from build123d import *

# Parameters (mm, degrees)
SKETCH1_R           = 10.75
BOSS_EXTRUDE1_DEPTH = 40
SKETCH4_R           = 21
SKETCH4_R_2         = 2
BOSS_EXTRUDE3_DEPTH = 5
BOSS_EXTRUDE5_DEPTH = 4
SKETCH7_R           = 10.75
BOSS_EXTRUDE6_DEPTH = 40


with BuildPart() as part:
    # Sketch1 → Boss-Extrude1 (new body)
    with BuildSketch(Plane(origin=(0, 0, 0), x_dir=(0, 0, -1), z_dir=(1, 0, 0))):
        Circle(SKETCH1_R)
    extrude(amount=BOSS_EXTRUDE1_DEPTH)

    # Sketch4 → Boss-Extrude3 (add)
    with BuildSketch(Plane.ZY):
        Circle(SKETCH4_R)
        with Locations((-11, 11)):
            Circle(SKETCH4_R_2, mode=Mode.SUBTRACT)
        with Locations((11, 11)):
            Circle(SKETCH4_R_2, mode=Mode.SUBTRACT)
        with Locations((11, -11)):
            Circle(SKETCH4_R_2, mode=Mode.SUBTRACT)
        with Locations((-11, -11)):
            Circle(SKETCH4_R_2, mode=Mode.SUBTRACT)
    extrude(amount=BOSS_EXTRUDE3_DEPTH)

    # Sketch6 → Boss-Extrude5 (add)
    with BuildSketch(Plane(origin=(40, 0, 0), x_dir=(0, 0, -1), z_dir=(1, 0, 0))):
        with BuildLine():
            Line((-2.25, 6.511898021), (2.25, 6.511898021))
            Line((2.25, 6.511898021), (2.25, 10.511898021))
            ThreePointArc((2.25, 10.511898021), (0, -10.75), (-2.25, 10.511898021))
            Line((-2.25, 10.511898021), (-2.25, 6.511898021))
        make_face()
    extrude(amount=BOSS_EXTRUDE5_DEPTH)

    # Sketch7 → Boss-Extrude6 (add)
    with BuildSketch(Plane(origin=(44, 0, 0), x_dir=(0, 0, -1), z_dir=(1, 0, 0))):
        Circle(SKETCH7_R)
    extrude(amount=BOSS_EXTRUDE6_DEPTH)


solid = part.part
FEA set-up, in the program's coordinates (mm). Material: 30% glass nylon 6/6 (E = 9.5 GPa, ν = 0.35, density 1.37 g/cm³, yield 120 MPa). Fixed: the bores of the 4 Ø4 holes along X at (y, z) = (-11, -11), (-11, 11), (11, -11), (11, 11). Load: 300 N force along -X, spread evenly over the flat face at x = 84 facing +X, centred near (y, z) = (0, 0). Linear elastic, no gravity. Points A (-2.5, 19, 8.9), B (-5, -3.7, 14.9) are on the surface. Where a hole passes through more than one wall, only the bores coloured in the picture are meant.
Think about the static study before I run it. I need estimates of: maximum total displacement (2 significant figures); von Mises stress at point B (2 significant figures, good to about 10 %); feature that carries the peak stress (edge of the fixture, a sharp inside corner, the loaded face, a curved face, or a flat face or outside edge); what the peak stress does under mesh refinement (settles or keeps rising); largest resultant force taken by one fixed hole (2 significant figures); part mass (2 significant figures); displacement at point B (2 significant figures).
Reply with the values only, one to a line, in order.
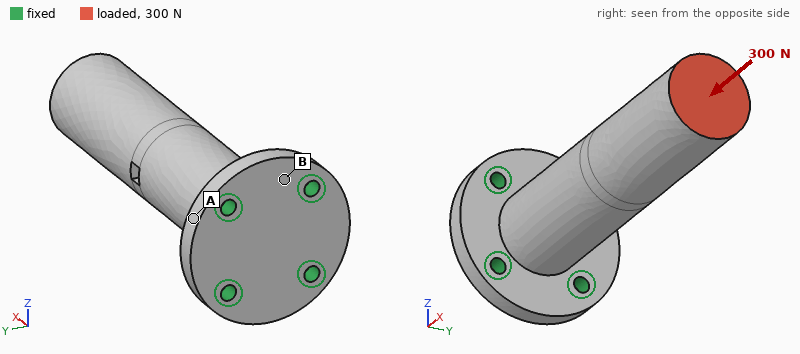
11 µm
0.91 MPa
edge of the fixture
keeps rising
78 N
51 g
1.7 µm
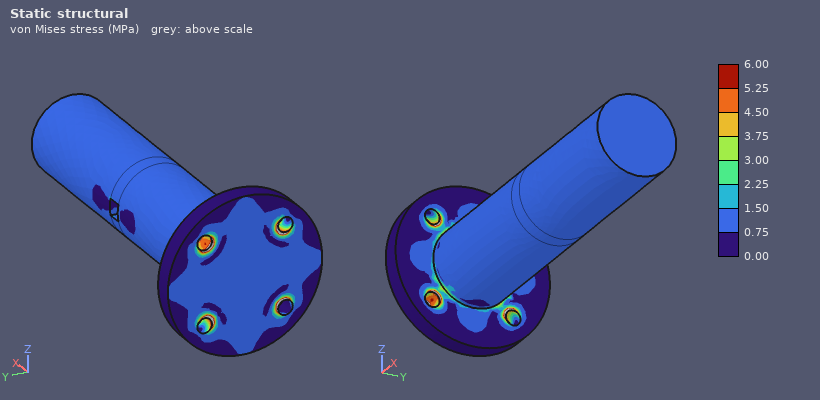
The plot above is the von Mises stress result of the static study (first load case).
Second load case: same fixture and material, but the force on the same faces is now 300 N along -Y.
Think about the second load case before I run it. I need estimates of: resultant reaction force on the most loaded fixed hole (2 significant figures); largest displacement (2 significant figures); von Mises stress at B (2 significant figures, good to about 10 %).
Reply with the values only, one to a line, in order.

650 N
0.93 mm
6.2 MPa
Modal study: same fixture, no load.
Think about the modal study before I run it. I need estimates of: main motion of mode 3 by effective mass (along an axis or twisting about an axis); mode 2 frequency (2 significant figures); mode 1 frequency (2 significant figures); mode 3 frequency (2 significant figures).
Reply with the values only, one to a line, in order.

twisting about X
850 Hz
850 Hz
4600 Hz
